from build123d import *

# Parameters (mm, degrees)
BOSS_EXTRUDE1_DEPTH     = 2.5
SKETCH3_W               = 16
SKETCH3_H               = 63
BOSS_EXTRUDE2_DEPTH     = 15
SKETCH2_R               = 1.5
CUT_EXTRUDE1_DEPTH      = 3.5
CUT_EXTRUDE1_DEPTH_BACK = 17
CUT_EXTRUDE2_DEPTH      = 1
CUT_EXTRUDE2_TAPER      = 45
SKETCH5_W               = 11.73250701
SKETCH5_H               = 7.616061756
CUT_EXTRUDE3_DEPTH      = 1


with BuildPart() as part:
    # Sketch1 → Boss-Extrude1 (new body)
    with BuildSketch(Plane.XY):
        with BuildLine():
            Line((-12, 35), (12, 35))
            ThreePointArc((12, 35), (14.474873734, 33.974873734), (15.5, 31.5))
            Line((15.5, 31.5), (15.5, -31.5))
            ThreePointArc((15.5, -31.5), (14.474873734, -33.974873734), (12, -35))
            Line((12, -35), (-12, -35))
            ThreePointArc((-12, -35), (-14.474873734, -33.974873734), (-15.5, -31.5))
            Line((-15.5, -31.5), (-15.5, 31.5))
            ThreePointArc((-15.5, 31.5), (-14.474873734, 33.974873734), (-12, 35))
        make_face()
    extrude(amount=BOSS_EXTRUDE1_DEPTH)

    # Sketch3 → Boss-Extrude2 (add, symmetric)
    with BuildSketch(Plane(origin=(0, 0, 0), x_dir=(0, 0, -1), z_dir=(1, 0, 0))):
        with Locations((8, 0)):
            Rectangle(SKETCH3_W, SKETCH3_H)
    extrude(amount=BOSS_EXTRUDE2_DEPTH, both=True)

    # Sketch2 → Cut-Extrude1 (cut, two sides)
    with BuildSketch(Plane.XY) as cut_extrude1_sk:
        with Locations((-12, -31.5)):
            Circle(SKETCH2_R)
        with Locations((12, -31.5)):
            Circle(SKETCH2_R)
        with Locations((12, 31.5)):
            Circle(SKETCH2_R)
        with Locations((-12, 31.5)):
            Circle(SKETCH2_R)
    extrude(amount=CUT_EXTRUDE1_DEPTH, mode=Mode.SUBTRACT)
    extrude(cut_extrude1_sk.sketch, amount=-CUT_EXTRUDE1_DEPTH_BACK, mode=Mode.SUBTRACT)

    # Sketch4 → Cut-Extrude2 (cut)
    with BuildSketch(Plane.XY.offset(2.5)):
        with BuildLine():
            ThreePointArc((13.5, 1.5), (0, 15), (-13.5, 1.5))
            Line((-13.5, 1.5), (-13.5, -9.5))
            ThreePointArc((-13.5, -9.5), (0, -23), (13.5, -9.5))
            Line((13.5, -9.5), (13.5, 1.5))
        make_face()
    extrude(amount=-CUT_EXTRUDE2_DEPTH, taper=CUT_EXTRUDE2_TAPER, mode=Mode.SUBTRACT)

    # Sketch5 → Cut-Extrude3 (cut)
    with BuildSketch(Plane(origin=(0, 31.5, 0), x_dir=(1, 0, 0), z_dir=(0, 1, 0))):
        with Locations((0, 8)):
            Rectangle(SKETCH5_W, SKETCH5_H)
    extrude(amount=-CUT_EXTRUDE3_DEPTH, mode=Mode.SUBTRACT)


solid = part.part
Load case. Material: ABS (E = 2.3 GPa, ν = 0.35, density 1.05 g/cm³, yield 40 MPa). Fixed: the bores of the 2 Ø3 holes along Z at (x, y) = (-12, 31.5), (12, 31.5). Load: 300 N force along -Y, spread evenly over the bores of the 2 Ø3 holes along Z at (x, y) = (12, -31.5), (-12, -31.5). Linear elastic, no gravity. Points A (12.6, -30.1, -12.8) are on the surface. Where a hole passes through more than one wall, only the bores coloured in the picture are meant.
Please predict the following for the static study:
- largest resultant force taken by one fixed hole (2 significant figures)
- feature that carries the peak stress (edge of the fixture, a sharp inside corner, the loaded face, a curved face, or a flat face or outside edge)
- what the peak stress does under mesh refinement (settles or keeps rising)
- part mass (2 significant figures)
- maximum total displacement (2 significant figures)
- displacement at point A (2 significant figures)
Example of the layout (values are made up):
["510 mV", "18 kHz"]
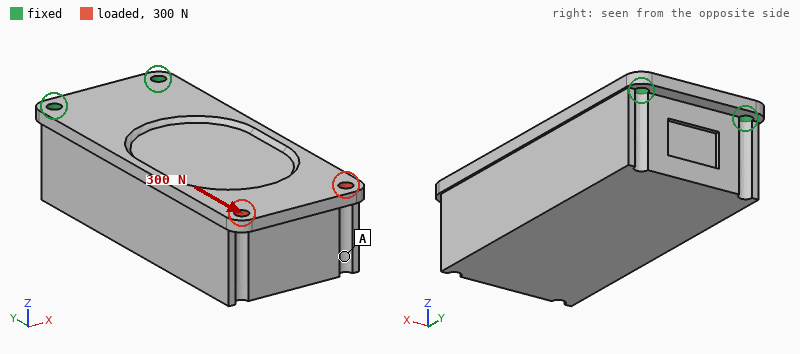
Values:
["150 N", "a sharp inside corner", "keeps rising", "36 g", "0.34 mm", "0.27 mm"]
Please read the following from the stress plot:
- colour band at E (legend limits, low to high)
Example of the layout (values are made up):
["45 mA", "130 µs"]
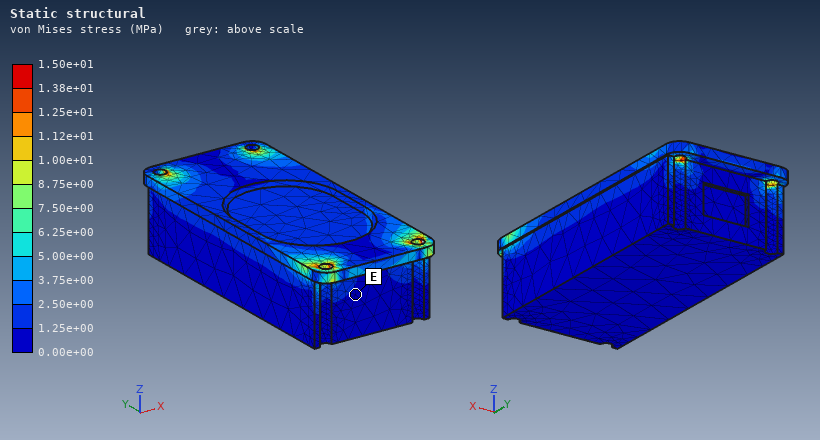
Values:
["0.00e+00 to 1.25e+00 MPa"]
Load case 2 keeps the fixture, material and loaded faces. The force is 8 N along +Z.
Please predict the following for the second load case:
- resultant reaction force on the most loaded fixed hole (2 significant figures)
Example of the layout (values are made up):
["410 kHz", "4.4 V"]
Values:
["4.0 N"]
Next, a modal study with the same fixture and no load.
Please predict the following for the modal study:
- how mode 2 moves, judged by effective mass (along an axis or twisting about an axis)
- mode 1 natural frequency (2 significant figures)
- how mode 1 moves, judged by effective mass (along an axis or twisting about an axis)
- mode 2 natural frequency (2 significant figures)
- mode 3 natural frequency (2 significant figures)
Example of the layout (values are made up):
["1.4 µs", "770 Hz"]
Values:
["along X", "150 Hz", "along Z", "930 Hz", "2200 Hz"]
